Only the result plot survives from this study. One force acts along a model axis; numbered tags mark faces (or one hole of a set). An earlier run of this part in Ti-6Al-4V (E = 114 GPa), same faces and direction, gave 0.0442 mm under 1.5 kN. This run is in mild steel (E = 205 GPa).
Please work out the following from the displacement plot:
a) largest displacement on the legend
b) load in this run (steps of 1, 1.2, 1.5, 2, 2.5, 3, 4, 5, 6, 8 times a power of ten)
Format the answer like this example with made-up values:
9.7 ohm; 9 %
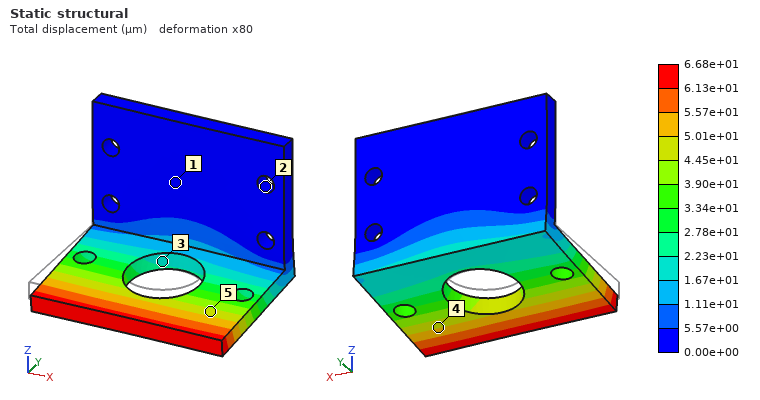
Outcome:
6.68e+01 µm; 4 kN
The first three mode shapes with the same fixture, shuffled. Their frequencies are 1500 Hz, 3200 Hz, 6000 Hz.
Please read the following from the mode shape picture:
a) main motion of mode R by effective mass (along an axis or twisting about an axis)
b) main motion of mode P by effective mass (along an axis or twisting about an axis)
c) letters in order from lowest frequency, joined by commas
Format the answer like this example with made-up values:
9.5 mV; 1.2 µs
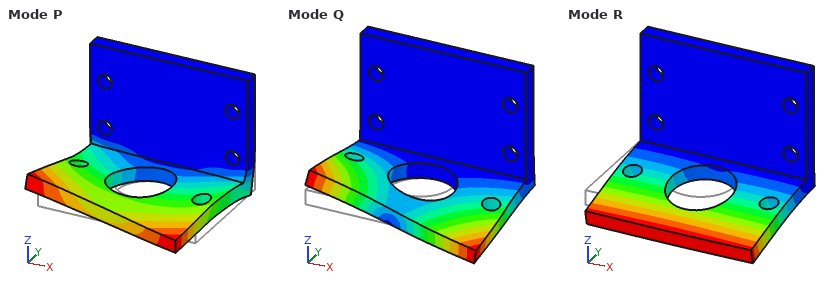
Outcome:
along Z; along X; R, Q, P
